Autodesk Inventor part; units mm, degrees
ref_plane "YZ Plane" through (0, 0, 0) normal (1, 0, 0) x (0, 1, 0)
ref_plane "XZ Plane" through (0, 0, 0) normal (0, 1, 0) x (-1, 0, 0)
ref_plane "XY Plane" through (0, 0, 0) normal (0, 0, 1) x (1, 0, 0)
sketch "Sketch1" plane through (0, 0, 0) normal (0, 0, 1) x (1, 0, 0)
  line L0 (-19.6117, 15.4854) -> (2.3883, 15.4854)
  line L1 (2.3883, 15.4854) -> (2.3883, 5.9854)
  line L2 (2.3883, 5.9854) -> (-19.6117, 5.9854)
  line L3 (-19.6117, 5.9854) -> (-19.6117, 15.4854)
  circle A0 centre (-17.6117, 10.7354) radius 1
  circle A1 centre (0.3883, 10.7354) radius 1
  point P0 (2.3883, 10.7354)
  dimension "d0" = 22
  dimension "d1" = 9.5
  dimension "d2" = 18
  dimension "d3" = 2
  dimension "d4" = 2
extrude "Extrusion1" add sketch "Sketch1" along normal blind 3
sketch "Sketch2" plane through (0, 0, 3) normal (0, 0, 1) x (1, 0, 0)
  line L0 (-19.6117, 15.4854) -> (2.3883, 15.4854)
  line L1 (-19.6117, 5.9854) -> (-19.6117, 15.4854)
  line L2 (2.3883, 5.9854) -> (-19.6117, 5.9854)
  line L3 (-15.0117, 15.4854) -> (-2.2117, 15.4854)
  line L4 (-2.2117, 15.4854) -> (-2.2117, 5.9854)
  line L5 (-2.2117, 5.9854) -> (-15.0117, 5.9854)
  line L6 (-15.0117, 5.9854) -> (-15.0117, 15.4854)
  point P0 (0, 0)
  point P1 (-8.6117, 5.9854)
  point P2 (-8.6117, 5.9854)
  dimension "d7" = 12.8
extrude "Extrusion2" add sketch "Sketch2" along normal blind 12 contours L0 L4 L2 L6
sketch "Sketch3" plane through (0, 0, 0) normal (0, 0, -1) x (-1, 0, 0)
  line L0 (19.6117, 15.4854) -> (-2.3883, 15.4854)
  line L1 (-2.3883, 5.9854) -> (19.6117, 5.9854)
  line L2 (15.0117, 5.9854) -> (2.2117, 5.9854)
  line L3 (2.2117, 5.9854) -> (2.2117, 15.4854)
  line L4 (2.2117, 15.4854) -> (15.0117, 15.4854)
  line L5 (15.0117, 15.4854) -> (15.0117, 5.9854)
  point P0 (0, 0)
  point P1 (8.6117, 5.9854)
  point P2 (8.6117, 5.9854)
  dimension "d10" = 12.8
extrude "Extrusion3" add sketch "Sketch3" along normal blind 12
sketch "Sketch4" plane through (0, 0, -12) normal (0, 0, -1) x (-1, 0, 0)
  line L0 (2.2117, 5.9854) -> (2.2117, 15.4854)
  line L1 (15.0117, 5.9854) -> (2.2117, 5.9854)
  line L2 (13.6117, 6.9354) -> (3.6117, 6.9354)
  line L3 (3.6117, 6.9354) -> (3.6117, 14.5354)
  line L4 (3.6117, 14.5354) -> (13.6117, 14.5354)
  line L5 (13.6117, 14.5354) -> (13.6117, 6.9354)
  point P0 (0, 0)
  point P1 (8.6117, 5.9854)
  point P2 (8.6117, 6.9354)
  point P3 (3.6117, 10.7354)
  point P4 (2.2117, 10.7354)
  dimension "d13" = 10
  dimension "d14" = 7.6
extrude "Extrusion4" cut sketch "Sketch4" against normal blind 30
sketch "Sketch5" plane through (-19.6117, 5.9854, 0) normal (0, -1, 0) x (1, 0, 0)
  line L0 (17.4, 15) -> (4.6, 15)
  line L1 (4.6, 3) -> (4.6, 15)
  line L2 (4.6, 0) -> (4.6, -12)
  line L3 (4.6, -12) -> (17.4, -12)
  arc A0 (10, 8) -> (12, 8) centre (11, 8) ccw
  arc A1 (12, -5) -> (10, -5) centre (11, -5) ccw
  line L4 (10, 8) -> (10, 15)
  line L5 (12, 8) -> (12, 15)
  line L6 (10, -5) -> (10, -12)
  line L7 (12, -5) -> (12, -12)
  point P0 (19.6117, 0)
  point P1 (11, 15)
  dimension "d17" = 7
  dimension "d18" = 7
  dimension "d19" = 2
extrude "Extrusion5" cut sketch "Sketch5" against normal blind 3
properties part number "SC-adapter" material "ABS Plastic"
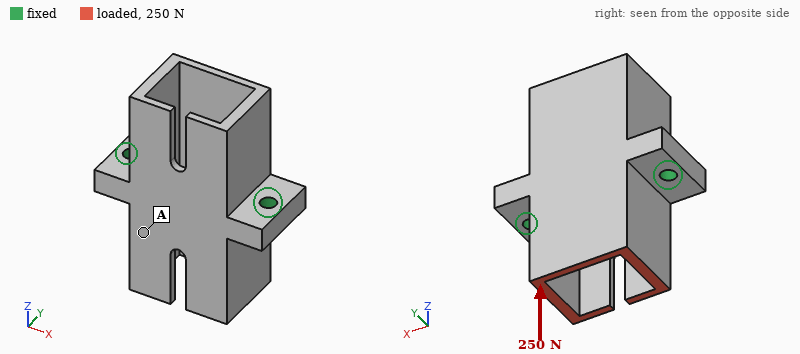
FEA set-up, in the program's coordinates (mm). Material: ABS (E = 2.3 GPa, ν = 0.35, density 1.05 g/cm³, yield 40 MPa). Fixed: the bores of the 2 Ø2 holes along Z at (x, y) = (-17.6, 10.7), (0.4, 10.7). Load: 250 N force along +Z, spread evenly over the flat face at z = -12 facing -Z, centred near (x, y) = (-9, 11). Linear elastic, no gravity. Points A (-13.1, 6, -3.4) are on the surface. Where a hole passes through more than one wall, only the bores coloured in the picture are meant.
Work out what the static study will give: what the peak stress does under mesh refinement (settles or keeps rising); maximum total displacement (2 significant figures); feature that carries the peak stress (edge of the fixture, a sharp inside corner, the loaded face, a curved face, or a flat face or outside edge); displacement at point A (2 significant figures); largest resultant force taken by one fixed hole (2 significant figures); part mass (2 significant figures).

keeps rising
89 µm
edge of the fixture
50 µm
130 N
1.5 g
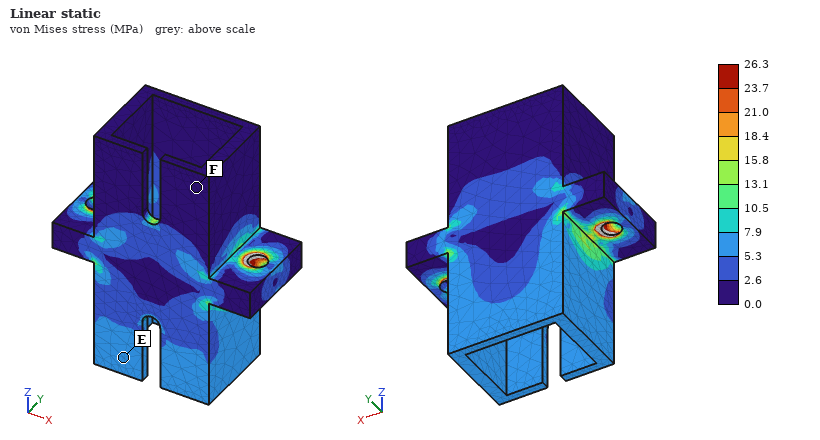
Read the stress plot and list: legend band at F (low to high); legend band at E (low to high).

0.0 to 2.6 MPa
5.3 to 7.9 MPa
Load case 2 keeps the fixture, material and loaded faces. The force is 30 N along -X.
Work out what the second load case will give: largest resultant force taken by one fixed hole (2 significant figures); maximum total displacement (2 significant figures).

31 N
0.10 mm
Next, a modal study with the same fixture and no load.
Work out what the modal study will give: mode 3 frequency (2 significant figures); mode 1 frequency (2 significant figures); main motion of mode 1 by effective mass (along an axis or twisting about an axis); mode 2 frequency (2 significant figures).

6400 Hz
3100 Hz
twisting about X
4900 Hz
